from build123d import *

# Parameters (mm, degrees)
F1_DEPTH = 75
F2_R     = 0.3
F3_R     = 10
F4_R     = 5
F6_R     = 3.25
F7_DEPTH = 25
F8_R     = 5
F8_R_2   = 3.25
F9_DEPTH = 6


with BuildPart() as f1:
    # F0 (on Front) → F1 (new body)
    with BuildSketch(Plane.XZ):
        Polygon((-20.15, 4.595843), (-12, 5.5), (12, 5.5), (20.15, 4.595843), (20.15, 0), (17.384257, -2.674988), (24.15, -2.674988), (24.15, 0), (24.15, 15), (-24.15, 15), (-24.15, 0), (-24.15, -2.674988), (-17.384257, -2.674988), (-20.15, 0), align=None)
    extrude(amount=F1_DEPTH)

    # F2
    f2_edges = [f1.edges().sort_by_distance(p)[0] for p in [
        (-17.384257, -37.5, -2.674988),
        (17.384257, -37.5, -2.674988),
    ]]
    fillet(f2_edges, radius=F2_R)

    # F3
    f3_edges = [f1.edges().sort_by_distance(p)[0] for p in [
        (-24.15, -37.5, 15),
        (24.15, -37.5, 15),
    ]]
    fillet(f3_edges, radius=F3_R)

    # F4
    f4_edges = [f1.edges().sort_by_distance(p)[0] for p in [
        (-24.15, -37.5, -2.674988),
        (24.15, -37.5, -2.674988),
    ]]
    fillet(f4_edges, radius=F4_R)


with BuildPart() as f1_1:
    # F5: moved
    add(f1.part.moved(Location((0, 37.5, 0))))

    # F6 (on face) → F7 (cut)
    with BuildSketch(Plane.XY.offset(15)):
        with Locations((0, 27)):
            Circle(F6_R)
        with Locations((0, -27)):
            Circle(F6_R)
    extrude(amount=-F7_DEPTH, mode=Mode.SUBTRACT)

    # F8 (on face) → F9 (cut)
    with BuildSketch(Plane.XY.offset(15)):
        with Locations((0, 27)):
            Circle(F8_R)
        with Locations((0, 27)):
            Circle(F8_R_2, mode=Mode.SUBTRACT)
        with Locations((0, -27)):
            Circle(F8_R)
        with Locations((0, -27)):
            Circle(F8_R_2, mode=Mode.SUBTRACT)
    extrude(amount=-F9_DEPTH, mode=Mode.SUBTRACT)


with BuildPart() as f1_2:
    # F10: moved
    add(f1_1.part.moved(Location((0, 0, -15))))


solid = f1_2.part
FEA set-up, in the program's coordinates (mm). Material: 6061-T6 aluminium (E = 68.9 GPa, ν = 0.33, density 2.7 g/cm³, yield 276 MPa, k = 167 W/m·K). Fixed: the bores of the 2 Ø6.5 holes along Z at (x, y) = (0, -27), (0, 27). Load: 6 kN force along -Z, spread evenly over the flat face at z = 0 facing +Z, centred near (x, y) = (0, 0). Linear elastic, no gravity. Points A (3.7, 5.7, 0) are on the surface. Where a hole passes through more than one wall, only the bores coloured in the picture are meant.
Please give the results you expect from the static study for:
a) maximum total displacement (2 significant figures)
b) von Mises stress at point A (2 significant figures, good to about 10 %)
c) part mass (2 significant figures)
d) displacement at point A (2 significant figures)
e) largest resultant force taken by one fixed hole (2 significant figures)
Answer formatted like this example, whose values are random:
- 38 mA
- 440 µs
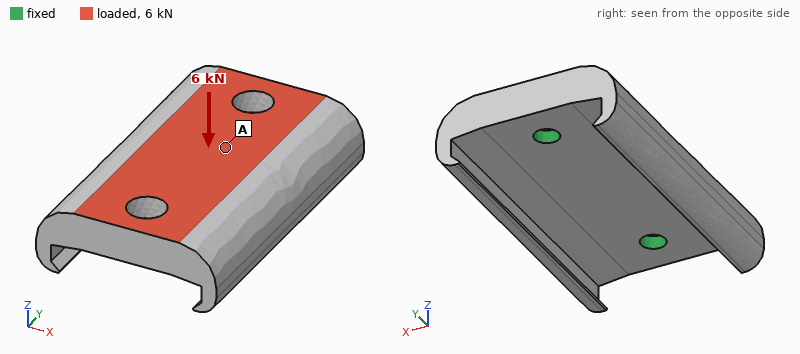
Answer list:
- 26 µm
- 22 MPa
- 95 g
- 22 µm
- 3.2 kN
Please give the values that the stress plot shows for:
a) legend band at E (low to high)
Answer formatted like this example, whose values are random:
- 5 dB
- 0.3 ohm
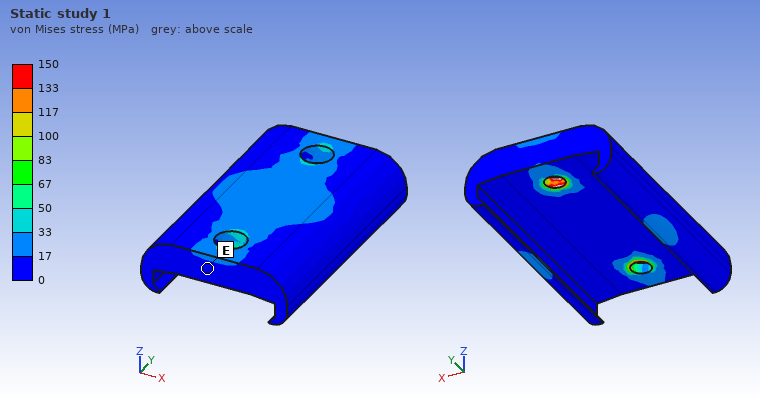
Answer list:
- 0 to 17 MPa
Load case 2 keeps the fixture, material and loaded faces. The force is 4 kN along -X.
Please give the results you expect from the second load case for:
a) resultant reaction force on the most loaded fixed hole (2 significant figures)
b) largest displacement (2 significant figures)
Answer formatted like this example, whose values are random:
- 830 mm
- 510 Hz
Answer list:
- 2.0 kN
- 66 µm
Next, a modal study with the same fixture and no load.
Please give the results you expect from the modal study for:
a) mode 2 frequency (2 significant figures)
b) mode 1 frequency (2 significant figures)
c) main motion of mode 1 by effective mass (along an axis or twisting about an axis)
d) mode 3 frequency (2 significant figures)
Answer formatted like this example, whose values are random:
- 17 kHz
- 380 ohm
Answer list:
- 7900 Hz
- 3700 Hz
- twisting about Y
- 8100 Hz
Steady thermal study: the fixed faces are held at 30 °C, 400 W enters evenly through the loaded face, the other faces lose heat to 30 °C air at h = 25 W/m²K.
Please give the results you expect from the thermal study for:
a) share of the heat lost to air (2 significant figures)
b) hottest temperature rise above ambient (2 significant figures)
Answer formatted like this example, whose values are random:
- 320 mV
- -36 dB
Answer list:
- 3.4 %
- 77 K
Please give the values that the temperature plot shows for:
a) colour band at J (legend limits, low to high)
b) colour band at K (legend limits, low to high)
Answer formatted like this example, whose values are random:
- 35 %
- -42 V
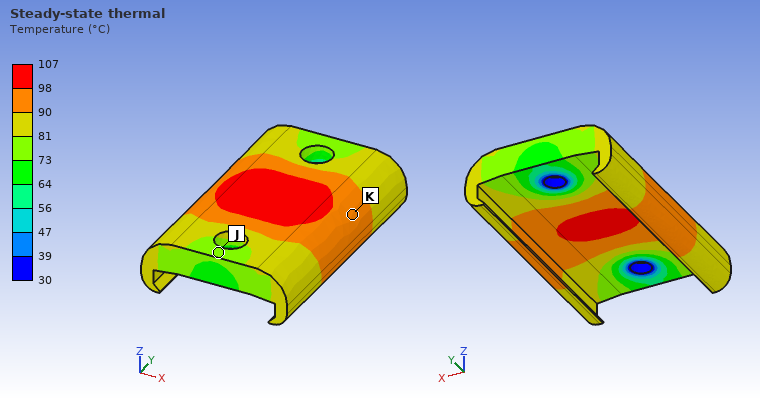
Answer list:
- 73 to 81 °C
- 90 to 98 °C
